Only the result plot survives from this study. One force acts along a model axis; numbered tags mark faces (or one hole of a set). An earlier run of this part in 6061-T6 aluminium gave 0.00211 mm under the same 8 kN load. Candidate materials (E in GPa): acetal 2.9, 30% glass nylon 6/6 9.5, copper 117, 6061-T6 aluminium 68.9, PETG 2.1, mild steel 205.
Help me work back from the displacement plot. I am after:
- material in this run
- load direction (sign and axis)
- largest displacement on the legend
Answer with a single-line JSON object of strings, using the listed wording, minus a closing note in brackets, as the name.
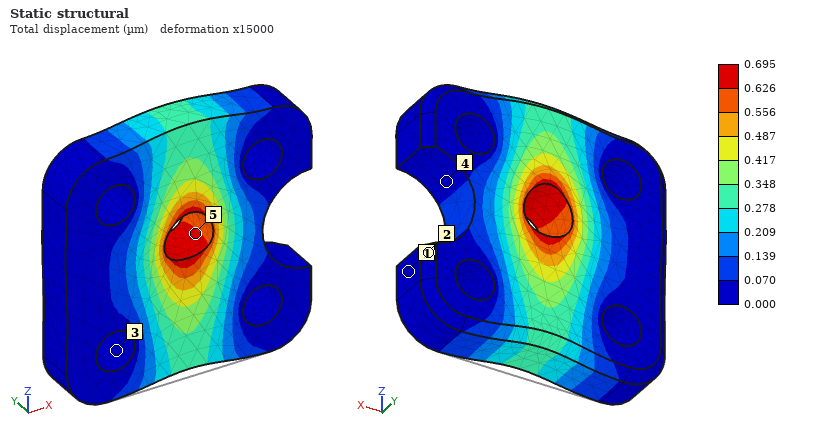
{"material in this run": "mild steel", "load direction": "+Z", "largest displacement on the legend": "0.695 µm"}
